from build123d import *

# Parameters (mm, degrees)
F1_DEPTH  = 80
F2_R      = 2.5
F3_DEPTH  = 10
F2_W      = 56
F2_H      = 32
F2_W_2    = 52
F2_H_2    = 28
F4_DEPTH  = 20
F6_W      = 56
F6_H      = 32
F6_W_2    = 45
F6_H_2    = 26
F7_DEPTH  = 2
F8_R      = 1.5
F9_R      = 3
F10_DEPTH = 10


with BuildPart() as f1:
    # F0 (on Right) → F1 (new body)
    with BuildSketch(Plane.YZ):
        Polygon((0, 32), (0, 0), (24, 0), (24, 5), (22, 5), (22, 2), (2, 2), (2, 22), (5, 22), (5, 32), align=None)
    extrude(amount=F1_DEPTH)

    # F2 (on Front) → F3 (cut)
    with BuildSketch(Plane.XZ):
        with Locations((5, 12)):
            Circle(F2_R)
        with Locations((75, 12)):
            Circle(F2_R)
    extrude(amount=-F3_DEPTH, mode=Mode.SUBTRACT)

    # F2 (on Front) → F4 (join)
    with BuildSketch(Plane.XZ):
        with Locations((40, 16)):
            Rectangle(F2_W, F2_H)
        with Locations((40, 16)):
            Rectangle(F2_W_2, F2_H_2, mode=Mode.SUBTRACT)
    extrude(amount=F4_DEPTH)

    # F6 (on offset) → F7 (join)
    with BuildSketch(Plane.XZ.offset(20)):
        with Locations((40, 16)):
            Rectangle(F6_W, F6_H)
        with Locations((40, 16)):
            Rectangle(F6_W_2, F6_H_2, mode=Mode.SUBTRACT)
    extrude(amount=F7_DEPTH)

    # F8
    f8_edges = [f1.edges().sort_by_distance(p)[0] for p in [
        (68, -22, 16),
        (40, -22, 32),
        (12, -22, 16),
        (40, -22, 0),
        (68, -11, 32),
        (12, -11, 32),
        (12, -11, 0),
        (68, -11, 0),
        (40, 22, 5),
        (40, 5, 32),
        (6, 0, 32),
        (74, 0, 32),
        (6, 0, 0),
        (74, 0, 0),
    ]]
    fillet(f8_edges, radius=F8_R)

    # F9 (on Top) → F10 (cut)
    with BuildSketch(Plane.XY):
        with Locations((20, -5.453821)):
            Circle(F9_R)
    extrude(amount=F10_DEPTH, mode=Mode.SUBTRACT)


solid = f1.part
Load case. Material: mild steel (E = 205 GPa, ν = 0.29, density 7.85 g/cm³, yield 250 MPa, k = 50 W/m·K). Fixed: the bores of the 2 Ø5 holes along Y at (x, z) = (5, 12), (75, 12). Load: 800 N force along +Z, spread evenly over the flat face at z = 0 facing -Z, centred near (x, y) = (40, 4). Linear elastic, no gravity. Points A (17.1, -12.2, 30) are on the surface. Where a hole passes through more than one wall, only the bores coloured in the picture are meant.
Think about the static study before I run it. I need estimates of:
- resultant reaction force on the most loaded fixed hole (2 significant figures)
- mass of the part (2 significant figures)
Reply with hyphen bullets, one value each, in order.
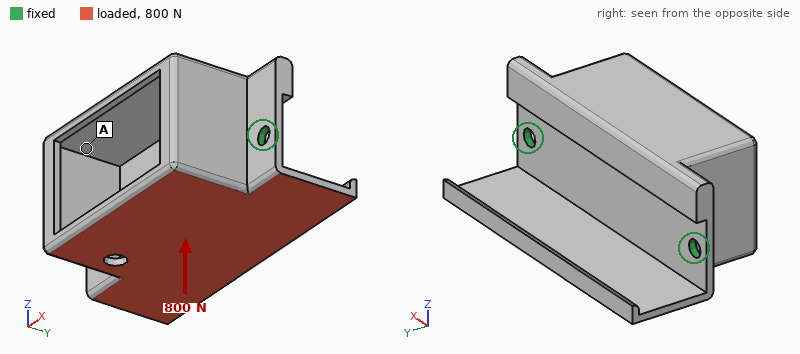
- 400 N
- 150 g
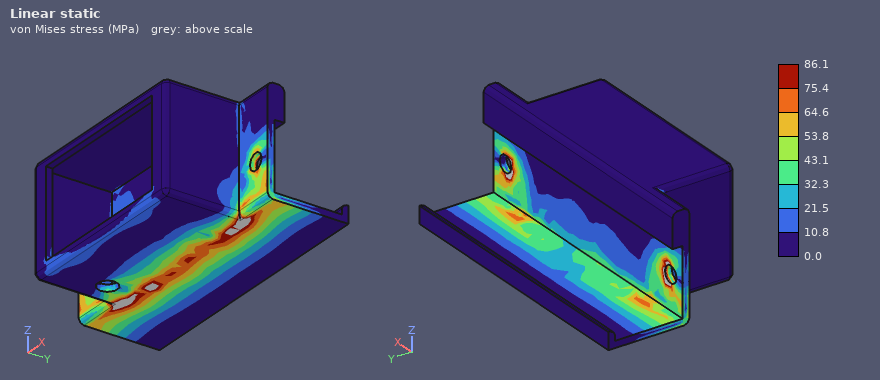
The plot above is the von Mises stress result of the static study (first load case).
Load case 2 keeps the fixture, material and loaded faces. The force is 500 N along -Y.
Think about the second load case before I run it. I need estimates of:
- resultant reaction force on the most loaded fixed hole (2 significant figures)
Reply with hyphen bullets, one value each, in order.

- 250 N
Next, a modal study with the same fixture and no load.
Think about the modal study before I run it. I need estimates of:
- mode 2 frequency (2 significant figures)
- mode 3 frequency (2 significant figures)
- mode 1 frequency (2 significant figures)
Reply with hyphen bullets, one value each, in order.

- 2700 Hz
- 2700 Hz
- 1400 Hz
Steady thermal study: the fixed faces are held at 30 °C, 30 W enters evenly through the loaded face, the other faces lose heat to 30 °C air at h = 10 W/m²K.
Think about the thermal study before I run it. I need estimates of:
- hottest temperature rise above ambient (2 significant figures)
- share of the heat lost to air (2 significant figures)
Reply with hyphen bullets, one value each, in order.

- 84 K
- 23 %
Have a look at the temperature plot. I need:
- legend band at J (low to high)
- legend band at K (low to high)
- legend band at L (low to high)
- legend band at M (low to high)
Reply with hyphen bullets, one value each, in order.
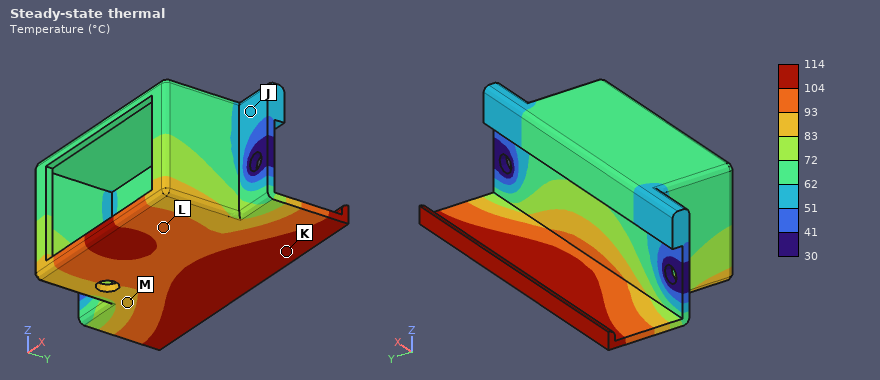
- 51 to 62 °C
- 104 to 114 °C
- 93 to 104 °C
- 83 to 93 °C
